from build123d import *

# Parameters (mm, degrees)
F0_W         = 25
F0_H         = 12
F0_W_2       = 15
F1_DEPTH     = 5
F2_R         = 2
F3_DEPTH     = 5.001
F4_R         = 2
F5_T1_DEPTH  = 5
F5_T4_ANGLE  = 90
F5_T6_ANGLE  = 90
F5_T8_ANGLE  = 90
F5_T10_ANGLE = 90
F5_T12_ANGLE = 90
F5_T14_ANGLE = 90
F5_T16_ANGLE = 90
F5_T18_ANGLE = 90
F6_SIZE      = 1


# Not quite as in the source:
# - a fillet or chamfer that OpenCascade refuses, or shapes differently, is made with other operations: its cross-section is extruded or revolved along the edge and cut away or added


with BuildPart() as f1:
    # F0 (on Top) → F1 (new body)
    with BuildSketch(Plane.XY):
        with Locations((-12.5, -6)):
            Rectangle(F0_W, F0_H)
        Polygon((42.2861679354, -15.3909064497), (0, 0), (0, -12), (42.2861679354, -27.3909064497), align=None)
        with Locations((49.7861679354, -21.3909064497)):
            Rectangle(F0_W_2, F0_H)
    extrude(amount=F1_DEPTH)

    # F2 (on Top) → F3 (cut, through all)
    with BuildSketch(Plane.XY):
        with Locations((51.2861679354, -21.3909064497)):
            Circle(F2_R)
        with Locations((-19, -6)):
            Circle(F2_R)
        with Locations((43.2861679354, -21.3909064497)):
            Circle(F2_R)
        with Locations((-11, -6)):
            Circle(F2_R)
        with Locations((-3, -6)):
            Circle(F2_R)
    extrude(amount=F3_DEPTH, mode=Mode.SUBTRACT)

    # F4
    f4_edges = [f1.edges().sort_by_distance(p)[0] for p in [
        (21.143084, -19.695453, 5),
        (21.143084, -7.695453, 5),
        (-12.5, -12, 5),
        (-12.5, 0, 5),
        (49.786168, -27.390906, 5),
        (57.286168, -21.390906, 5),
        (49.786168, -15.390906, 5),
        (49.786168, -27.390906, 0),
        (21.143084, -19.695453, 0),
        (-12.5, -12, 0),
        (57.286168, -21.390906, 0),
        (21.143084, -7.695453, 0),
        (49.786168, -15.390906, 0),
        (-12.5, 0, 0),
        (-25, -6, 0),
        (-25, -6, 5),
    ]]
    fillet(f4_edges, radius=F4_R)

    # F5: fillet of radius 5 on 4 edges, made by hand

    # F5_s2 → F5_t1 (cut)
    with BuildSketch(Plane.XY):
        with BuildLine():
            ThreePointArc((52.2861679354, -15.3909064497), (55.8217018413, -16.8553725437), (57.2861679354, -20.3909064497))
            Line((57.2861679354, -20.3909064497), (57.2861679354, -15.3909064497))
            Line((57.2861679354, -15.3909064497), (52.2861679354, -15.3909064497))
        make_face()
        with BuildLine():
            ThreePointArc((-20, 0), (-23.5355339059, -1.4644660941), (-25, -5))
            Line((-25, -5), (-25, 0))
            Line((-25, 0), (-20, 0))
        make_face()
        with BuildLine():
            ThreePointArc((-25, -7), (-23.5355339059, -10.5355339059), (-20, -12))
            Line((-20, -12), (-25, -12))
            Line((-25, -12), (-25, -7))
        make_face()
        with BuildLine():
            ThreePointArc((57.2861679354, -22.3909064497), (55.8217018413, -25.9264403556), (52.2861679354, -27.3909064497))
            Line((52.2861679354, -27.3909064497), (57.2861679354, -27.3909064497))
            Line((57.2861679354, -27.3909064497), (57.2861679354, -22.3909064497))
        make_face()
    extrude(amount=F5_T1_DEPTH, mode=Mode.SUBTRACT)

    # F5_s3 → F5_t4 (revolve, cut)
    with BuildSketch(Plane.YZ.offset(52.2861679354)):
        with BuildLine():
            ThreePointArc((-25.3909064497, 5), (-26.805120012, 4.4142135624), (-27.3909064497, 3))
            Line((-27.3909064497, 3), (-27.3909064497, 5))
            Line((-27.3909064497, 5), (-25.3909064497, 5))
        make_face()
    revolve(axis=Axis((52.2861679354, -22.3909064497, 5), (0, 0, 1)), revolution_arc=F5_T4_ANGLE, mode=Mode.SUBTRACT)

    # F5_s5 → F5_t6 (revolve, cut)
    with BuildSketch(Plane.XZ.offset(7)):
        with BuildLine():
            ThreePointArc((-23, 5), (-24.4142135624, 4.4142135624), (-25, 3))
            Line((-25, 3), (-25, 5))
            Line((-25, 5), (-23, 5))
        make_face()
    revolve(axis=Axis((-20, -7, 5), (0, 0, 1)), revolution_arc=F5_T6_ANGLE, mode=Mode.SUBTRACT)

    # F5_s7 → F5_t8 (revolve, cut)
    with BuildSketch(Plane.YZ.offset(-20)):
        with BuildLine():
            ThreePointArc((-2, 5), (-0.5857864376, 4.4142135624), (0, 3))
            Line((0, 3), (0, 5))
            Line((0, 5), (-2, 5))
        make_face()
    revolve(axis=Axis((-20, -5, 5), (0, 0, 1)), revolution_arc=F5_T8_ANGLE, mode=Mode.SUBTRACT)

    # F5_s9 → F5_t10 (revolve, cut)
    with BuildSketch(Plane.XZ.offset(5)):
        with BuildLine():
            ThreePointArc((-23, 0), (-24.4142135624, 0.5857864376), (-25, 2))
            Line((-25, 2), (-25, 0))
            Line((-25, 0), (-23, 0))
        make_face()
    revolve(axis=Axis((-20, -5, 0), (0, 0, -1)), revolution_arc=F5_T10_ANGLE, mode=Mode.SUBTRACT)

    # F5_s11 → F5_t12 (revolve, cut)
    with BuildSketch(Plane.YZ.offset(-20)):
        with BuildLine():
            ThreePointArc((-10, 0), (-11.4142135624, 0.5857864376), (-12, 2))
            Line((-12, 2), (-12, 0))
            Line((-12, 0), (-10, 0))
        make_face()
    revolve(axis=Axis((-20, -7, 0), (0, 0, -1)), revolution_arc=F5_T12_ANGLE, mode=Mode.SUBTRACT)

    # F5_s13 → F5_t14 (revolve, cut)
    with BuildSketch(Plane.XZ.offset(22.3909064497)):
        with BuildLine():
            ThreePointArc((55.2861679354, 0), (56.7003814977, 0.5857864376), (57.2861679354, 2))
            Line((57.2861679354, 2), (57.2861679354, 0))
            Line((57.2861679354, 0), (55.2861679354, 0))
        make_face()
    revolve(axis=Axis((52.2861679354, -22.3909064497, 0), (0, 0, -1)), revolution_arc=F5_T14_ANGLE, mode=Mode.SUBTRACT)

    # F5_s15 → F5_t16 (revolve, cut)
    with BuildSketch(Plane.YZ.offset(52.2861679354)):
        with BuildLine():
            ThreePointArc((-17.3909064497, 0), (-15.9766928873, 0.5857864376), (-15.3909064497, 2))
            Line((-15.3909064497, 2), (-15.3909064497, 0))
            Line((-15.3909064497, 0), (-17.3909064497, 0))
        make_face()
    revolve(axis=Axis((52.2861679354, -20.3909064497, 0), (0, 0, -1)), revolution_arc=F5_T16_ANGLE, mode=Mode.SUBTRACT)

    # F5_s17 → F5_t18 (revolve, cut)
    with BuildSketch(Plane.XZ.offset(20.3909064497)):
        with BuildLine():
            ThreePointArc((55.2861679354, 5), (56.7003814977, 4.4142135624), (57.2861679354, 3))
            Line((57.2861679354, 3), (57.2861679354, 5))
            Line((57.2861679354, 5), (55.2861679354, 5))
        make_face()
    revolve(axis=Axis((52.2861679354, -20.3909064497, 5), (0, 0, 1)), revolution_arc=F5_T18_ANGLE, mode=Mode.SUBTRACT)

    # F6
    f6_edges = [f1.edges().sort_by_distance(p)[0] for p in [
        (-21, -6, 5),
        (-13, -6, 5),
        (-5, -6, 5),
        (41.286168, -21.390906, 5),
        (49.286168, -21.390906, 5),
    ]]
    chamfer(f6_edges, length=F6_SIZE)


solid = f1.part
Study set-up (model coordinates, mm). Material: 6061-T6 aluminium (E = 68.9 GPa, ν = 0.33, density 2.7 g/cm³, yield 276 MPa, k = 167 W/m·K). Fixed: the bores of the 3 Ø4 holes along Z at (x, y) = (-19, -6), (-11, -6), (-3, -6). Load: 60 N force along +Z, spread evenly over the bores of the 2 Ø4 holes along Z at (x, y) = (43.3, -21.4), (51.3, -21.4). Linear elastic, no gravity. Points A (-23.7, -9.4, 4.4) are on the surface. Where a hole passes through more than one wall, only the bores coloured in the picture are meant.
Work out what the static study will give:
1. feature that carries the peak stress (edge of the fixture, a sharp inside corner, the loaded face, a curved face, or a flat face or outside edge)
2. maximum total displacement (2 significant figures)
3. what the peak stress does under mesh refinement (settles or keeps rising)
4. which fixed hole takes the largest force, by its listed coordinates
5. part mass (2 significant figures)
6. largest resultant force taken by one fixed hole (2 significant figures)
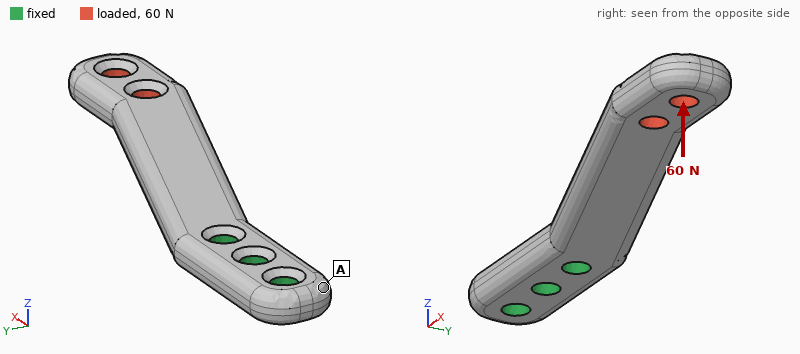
edge of the fixture
0.52 mm
keeps rising
(-3, -6)
11 g
140 N
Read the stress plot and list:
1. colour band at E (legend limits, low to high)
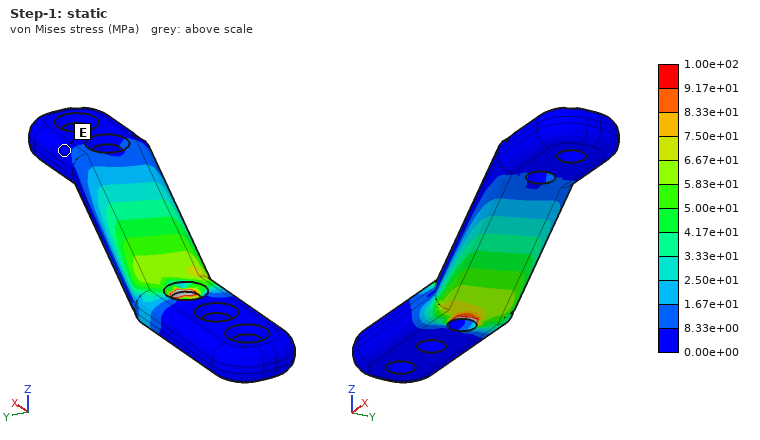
0.00e+00 to 8.33e+00 MPa
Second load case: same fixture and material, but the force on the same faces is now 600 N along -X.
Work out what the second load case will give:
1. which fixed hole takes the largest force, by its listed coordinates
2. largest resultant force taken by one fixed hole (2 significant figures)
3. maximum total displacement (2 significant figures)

(-3, -6)
650 N
0.36 mm
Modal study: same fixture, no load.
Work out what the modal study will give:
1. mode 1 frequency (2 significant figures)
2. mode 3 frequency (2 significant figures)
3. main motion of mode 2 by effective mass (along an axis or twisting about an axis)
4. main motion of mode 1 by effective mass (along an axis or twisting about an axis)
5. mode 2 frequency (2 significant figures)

1100 Hz
6300 Hz
along Y
along Z
2200 Hz
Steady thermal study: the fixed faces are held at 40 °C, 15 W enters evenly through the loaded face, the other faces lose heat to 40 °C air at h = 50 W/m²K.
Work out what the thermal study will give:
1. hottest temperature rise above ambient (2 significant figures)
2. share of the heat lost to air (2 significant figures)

76 K
24 %
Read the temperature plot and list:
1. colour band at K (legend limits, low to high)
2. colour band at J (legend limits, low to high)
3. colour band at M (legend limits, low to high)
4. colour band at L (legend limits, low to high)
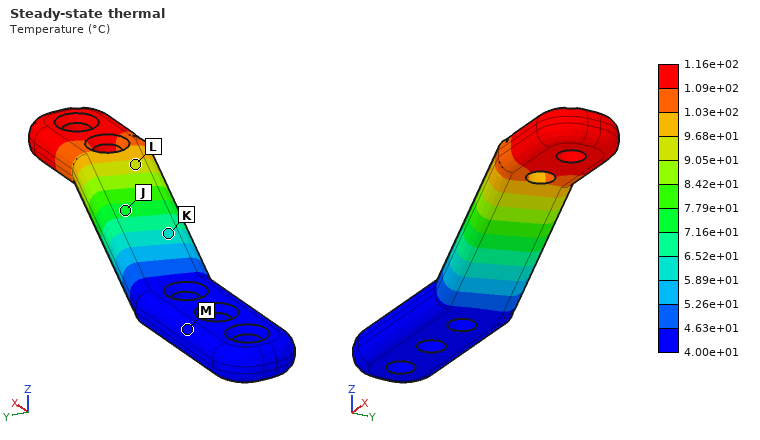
5.89e+01 to 6.52e+01 °C
7.16e+01 to 7.79e+01 °C
4.00e+01 to 4.63e+01 °C
9.05e+01 to 9.68e+01 °C
